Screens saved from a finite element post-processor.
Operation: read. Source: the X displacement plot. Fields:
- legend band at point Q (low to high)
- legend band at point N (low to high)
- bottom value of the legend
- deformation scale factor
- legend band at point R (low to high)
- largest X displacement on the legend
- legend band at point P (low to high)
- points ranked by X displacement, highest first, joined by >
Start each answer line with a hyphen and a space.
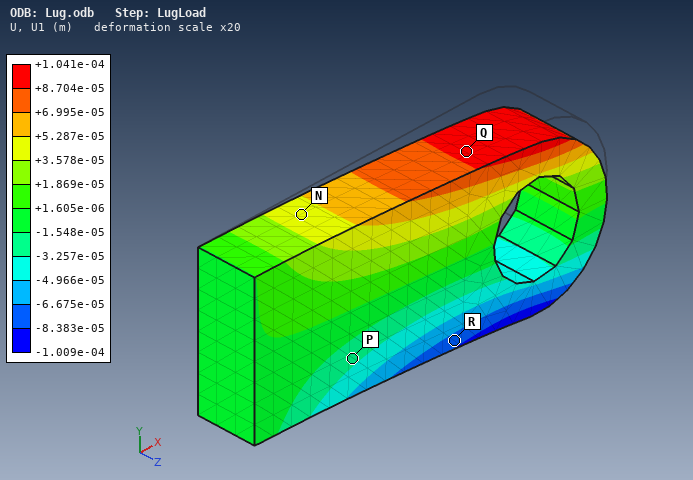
- +8.704e-05 to +1.041e-04 m
- +3.578e-05 to +5.287e-05 m
- -1.009e-04 m
- 20
- -8.383e-05 to -6.675e-05 m
- +1.041e-04 m
- -3.257e-05 to -1.548e-05 m
- Q > N > P > R
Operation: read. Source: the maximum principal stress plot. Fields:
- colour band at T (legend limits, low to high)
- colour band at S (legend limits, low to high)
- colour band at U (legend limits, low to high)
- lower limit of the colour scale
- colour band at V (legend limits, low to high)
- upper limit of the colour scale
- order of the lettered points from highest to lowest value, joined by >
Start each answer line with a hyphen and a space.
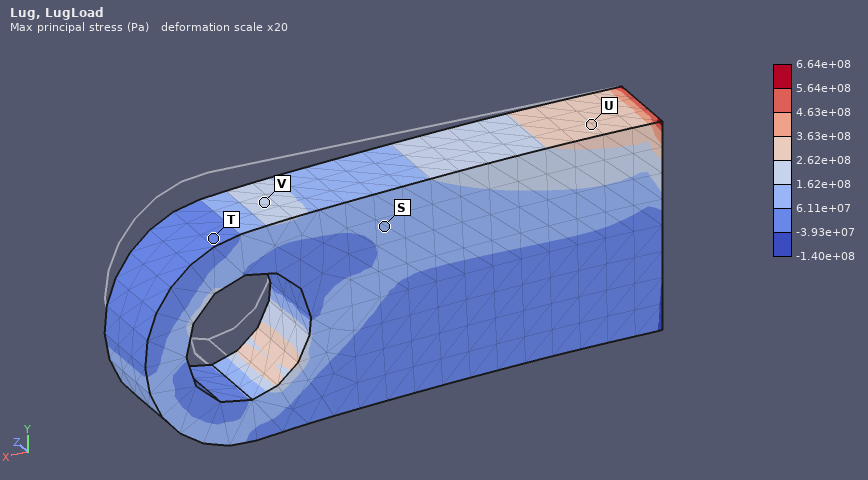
- -3.93e+07 to 6.11e+07 Pa
- 6.11e+07 to 1.62e+08 Pa
- 2.62e+08 to 3.63e+08 Pa
- -1.40e+08 Pa
- 1.62e+08 to 2.62e+08 Pa
- 6.64e+08 Pa
- U > V > S > T
